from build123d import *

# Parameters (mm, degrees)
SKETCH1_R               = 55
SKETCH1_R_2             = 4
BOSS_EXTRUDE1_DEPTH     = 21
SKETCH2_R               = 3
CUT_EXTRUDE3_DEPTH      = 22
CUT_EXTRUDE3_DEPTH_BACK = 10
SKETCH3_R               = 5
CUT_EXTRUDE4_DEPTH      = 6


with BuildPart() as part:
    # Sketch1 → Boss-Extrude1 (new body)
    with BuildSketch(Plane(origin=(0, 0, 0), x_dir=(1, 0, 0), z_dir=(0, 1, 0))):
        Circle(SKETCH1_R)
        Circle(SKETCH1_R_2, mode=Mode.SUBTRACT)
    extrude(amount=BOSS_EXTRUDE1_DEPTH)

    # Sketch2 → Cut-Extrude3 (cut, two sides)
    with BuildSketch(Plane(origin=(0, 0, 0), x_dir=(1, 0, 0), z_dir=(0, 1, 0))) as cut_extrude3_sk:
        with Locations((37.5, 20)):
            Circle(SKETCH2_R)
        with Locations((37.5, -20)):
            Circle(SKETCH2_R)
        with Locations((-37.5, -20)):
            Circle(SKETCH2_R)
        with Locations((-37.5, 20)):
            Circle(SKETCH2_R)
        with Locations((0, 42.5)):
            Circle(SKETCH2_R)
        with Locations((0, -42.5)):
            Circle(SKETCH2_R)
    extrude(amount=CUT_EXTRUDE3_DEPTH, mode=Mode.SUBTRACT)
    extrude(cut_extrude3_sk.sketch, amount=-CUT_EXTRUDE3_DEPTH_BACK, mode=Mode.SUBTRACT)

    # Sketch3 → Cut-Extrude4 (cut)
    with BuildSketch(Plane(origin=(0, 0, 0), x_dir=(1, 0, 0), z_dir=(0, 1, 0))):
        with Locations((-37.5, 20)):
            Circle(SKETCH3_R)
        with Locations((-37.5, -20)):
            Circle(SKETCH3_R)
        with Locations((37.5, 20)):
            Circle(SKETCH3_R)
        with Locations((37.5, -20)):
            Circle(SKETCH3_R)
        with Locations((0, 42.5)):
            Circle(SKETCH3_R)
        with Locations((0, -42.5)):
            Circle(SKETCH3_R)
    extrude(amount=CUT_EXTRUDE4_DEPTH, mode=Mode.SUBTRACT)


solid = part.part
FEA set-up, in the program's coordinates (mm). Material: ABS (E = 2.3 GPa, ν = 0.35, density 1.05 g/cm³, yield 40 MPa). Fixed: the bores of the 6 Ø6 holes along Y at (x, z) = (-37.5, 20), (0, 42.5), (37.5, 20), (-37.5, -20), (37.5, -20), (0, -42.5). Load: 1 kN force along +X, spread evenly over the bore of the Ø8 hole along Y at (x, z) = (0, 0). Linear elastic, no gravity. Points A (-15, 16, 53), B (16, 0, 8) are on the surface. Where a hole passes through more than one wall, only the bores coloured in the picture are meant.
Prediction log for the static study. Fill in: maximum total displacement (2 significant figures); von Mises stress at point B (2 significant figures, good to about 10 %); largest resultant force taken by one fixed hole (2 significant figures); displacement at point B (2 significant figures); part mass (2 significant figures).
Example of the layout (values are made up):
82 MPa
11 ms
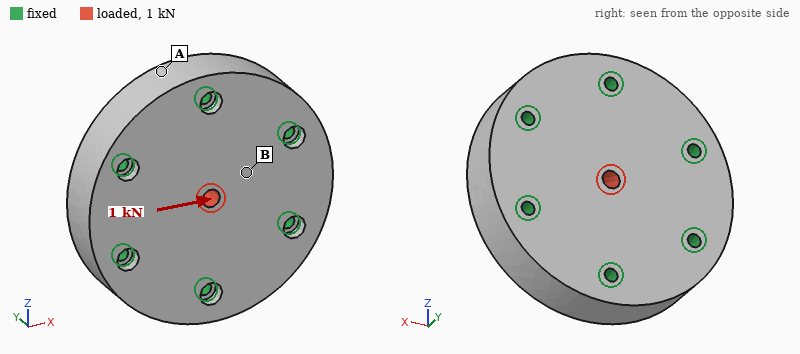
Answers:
16 µm
0.69 MPa
220 N
7.4 µm
200 g
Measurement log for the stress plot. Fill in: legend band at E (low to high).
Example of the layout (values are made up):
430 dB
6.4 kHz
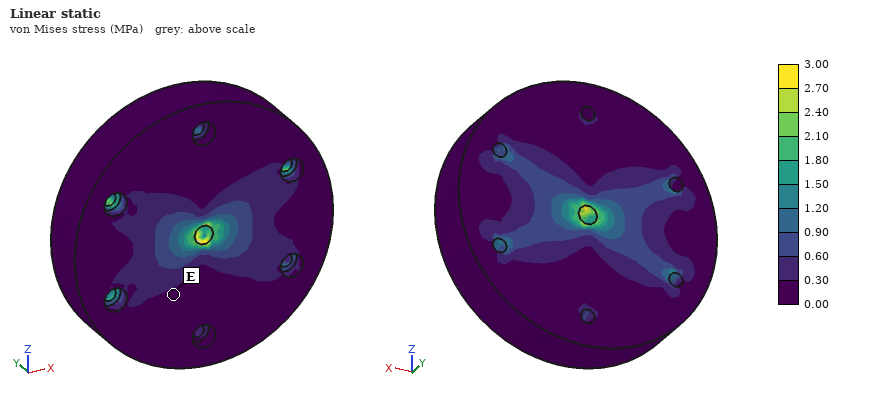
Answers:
0.00 to 0.30 MPa
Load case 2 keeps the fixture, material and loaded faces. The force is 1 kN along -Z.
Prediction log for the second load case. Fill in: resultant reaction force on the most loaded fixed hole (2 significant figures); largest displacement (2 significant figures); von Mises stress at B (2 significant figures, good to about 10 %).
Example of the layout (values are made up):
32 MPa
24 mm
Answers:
260 N
16 µm
0.39 MPa
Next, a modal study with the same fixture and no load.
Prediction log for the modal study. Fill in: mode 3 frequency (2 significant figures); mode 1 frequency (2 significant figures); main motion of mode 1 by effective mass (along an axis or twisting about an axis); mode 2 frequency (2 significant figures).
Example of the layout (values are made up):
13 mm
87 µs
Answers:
5900 Hz
4200 Hz
along Y
5800 Hz
